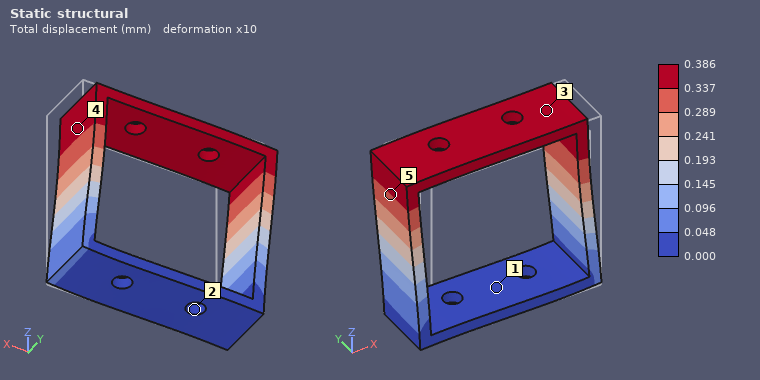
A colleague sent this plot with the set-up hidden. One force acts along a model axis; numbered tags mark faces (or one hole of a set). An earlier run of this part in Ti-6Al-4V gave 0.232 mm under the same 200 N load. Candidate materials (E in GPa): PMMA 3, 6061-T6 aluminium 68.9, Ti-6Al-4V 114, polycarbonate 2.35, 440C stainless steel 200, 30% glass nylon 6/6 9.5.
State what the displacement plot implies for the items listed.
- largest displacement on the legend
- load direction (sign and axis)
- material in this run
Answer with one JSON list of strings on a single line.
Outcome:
["0.386 mm", "-X", "6061-T6 aluminium"]
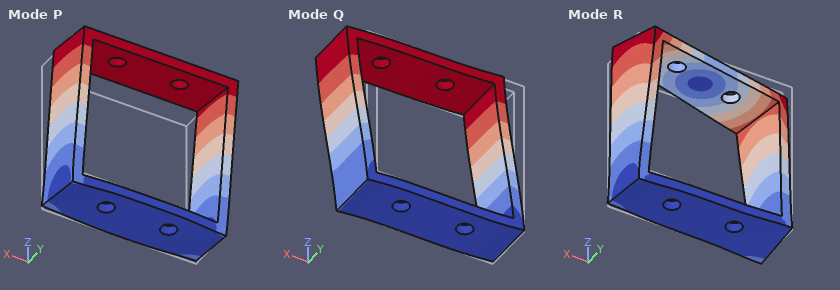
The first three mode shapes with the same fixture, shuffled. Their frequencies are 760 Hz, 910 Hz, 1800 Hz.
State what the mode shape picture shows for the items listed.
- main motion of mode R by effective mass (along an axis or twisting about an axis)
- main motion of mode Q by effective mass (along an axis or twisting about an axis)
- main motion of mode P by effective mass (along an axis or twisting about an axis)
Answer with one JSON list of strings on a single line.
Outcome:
["twisting about Z", "along X", "along Y"]
